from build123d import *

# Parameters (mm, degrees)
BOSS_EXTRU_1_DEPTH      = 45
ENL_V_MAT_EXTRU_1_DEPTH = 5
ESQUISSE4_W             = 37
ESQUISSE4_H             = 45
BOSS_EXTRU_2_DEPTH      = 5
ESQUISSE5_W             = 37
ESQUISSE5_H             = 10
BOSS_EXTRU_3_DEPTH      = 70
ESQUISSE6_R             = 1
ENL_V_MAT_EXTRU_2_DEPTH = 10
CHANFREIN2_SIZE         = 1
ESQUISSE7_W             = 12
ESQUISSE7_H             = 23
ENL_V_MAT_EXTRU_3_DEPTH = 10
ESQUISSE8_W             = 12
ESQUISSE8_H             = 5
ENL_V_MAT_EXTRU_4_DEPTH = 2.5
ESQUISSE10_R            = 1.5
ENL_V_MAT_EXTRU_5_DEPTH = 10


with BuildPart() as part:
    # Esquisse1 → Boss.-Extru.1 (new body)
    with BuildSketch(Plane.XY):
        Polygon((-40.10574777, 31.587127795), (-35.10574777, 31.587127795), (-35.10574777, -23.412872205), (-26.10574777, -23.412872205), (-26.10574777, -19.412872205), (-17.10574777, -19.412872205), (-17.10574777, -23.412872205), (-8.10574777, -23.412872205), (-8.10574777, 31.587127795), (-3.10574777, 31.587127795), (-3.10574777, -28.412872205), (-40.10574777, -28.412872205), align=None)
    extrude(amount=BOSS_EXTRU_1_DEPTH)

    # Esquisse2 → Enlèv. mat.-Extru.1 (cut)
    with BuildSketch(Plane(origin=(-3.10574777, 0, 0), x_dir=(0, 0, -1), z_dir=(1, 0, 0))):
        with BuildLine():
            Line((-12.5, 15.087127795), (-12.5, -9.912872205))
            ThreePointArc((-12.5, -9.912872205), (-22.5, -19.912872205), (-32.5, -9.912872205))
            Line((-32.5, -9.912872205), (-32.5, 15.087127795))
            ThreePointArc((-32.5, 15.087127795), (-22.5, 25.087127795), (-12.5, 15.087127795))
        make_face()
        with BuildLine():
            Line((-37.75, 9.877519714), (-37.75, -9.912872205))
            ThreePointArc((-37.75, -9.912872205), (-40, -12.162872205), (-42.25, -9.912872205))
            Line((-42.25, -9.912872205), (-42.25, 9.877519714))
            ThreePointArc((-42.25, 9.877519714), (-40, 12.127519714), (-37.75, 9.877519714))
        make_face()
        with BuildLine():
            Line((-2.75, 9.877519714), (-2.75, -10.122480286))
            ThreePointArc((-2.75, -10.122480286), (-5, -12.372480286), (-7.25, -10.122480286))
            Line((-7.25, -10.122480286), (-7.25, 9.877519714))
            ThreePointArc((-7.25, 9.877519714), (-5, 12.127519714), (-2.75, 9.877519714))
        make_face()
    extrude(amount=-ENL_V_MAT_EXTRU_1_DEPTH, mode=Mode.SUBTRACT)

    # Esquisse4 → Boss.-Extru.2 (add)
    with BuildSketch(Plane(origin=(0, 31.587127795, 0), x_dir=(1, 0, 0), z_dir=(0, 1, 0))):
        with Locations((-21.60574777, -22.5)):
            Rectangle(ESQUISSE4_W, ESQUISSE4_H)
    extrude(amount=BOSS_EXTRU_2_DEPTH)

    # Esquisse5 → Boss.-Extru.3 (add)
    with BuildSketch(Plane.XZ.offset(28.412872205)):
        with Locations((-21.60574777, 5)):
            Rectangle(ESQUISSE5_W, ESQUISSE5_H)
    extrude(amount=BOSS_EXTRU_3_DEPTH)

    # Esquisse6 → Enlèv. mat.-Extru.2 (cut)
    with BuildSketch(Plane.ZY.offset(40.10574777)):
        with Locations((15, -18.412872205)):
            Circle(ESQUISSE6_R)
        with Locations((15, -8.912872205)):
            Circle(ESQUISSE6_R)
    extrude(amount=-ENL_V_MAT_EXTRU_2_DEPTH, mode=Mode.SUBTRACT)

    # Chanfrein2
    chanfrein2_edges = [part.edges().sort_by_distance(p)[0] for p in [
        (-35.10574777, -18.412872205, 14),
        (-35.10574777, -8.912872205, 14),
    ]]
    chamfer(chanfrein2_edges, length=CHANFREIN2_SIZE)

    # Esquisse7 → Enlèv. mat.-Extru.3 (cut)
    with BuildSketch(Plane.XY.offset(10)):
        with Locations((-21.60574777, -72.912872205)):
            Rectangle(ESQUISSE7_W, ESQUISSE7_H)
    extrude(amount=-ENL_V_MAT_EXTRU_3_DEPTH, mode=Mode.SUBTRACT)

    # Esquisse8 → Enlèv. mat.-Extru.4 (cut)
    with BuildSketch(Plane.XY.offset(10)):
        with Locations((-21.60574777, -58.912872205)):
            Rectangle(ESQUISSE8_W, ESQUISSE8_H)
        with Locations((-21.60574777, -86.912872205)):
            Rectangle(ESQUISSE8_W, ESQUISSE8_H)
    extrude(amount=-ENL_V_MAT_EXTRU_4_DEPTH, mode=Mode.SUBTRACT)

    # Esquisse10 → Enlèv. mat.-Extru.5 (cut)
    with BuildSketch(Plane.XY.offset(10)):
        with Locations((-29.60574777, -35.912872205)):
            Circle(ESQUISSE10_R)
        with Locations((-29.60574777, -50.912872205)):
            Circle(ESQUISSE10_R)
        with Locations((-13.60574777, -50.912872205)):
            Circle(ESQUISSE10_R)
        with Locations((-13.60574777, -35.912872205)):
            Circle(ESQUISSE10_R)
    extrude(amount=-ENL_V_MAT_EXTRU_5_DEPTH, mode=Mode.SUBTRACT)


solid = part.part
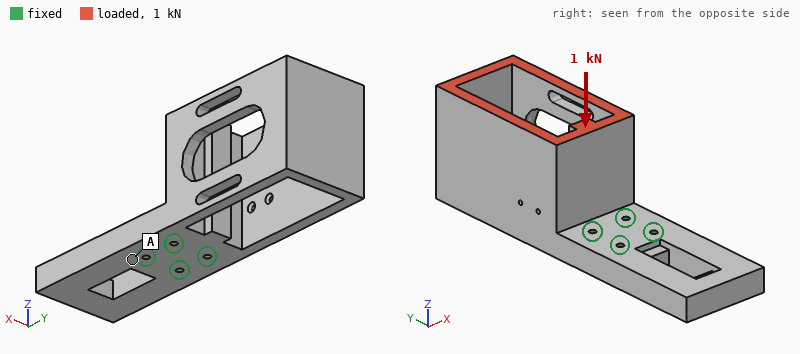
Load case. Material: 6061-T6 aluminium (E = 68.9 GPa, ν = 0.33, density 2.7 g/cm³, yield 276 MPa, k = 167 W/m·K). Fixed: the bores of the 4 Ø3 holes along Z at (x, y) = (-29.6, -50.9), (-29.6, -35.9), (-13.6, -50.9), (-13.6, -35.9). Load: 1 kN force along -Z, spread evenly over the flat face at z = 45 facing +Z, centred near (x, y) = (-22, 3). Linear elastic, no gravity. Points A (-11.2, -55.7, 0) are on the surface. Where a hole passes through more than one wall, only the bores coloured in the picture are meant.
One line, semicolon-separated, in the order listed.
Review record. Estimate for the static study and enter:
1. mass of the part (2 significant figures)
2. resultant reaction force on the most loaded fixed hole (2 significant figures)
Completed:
160 g; 950 N
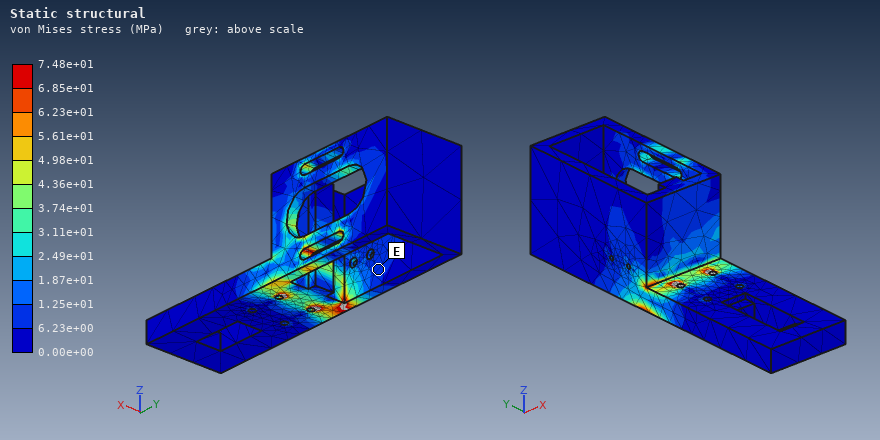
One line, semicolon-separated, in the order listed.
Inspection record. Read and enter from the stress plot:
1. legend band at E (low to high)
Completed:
6.23e+00 to 1.25e+01 MPa
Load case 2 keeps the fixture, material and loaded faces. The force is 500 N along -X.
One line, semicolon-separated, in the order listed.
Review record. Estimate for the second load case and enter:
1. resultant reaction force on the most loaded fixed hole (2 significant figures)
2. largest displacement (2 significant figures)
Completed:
1.1 kN; 0.16 mm
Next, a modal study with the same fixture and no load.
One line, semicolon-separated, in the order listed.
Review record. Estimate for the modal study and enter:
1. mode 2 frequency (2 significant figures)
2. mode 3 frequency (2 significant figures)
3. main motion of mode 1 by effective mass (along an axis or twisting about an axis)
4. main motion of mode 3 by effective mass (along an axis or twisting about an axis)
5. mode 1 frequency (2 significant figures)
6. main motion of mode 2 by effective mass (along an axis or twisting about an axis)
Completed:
1100 Hz; 2200 Hz; along Z; twisting about Y; 1000 Hz; along X
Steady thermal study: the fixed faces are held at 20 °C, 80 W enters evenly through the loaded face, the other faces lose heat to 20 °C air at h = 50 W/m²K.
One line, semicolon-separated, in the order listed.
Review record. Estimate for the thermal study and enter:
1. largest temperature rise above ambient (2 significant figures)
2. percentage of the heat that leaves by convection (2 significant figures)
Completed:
70 K; 37 %
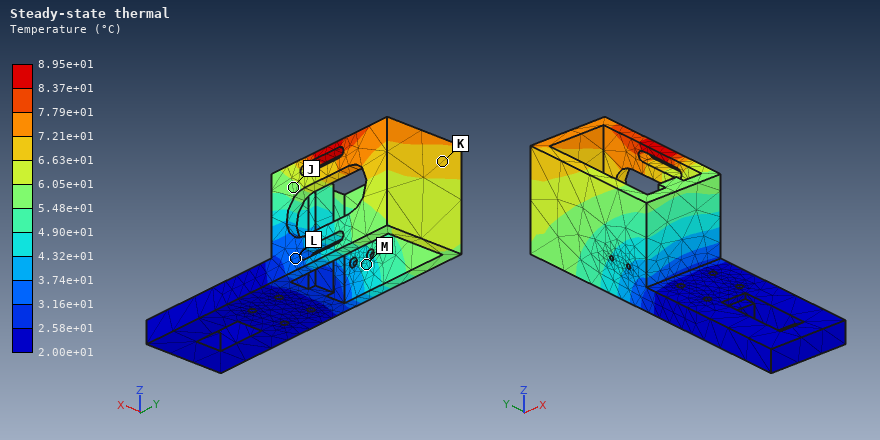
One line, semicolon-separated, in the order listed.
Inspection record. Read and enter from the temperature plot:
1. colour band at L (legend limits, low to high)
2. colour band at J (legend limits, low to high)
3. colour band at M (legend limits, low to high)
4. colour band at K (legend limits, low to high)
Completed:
3.16e+01 to 3.74e+01 °C; 5.48e+01 to 6.05e+01 °C; 4.32e+01 to 4.90e+01 °C; 6.63e+01 to 7.21e+01 °C
